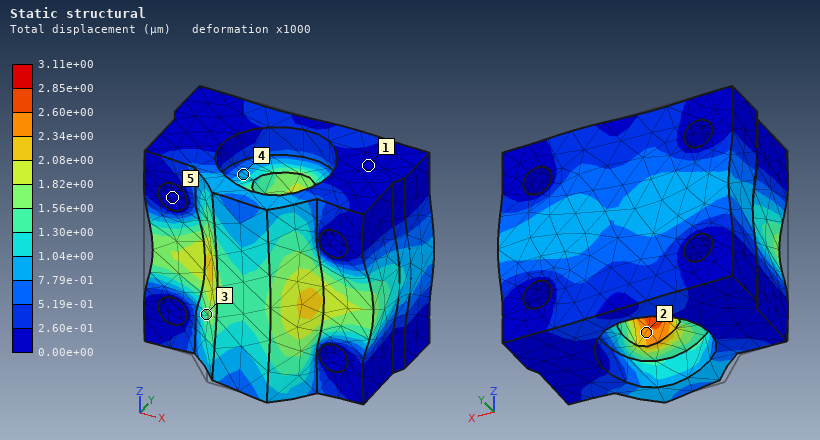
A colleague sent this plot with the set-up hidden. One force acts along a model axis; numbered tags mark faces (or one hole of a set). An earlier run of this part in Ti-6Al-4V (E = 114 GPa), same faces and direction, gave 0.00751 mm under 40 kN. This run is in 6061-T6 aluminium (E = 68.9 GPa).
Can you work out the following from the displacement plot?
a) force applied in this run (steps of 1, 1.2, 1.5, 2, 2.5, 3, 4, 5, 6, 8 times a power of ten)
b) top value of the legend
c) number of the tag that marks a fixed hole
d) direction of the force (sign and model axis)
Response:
10 kN
3.11e+00 µm
5
+X
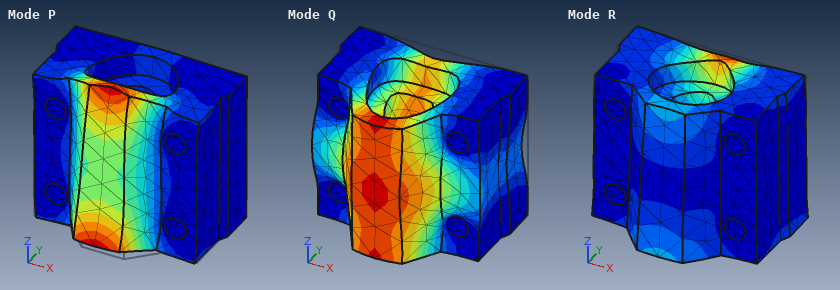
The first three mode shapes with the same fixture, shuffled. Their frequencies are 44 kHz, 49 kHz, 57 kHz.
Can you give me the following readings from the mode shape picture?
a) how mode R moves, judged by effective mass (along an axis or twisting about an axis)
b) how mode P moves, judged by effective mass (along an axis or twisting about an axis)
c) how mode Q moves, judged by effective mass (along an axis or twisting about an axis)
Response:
along Z
along Z
along Y
